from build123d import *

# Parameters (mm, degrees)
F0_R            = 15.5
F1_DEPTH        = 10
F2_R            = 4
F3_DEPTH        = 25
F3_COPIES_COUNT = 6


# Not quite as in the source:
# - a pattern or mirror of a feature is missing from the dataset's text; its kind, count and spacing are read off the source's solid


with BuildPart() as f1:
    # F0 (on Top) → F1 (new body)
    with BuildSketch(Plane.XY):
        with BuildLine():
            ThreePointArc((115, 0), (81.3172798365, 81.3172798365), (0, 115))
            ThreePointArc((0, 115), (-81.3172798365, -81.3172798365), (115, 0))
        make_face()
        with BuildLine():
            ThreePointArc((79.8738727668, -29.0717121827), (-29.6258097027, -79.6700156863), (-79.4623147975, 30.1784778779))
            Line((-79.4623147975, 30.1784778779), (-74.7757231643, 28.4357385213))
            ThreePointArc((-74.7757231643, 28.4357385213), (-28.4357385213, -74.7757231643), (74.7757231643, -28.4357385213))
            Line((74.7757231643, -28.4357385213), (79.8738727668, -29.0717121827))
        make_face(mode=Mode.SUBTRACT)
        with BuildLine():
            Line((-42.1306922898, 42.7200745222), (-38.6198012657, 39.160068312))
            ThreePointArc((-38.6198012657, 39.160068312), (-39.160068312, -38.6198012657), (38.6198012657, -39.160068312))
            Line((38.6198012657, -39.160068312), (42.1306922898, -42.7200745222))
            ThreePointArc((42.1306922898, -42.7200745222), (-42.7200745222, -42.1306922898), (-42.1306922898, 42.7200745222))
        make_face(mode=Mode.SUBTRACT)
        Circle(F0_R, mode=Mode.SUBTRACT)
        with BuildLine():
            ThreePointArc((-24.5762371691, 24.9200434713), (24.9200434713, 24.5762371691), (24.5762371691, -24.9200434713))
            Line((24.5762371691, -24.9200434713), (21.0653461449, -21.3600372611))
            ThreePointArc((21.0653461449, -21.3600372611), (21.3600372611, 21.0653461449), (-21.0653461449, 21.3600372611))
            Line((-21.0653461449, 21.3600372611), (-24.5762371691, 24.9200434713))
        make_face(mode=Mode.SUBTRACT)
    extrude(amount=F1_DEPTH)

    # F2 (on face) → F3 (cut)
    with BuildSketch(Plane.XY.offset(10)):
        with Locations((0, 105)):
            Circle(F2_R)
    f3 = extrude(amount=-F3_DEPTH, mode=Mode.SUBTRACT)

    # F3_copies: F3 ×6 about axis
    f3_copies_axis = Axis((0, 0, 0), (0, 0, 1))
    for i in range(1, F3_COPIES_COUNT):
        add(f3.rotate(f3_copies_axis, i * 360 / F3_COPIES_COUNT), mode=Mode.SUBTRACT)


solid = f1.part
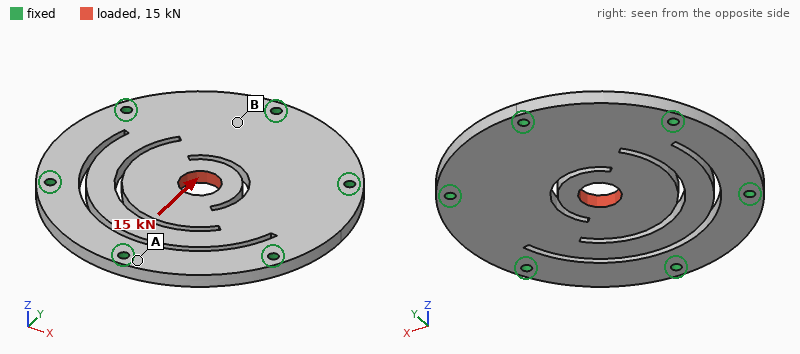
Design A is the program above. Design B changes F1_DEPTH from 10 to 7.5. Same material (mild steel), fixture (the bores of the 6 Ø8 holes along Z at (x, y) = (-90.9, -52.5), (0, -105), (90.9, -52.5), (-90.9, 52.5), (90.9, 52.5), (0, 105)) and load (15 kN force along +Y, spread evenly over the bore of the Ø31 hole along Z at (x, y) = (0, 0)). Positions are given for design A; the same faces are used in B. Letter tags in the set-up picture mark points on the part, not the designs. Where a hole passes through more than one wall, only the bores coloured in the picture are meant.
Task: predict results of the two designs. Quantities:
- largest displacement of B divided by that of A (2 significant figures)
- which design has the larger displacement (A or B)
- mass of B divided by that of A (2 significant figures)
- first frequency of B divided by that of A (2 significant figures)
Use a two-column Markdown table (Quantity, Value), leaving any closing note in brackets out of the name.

| Quantity | Value |
|---|---|
| largest displacement of B divided by that of A | 1.3 |
| which design has the larger displacement | B |
| mass of B divided by that of A | 0.75 |
| first frequency of B divided by that of A | 0.77 |
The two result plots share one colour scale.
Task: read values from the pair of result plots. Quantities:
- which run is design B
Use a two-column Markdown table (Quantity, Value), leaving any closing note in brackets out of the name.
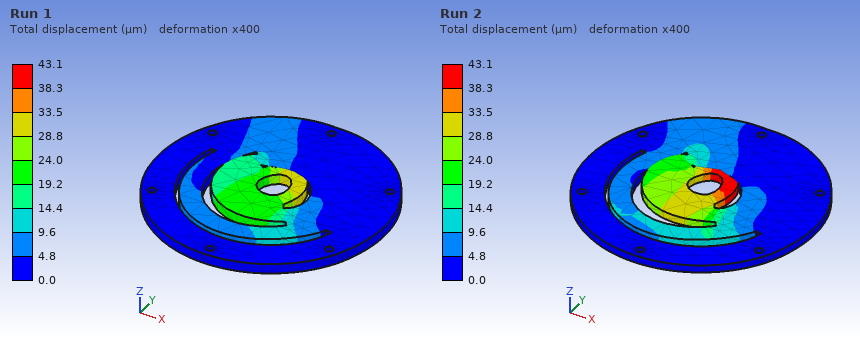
| Quantity | Value |
|---|---|
| which run is design B | Run 2 |
